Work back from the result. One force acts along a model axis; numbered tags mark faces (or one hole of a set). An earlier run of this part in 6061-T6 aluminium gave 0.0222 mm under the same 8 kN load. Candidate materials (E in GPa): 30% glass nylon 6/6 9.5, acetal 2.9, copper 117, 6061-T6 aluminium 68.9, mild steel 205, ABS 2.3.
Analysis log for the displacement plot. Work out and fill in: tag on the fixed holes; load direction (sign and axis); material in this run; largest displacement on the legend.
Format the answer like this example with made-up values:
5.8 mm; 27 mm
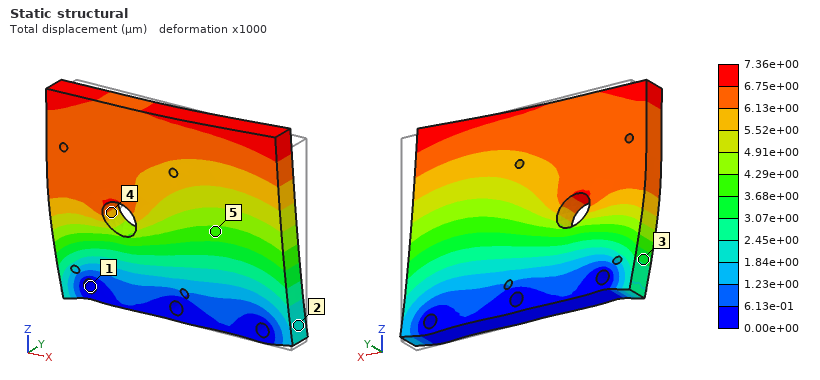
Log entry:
1; -X; mild steel; 7.36e+00 µm
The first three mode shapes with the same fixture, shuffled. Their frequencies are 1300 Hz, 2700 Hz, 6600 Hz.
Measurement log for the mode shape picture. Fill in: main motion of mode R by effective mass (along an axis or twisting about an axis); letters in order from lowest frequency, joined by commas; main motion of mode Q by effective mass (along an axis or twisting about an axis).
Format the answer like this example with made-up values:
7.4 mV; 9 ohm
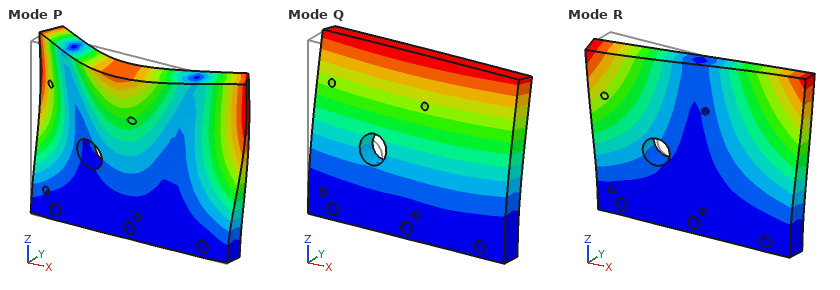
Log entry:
twisting about Z; Q, R, P; along Y
